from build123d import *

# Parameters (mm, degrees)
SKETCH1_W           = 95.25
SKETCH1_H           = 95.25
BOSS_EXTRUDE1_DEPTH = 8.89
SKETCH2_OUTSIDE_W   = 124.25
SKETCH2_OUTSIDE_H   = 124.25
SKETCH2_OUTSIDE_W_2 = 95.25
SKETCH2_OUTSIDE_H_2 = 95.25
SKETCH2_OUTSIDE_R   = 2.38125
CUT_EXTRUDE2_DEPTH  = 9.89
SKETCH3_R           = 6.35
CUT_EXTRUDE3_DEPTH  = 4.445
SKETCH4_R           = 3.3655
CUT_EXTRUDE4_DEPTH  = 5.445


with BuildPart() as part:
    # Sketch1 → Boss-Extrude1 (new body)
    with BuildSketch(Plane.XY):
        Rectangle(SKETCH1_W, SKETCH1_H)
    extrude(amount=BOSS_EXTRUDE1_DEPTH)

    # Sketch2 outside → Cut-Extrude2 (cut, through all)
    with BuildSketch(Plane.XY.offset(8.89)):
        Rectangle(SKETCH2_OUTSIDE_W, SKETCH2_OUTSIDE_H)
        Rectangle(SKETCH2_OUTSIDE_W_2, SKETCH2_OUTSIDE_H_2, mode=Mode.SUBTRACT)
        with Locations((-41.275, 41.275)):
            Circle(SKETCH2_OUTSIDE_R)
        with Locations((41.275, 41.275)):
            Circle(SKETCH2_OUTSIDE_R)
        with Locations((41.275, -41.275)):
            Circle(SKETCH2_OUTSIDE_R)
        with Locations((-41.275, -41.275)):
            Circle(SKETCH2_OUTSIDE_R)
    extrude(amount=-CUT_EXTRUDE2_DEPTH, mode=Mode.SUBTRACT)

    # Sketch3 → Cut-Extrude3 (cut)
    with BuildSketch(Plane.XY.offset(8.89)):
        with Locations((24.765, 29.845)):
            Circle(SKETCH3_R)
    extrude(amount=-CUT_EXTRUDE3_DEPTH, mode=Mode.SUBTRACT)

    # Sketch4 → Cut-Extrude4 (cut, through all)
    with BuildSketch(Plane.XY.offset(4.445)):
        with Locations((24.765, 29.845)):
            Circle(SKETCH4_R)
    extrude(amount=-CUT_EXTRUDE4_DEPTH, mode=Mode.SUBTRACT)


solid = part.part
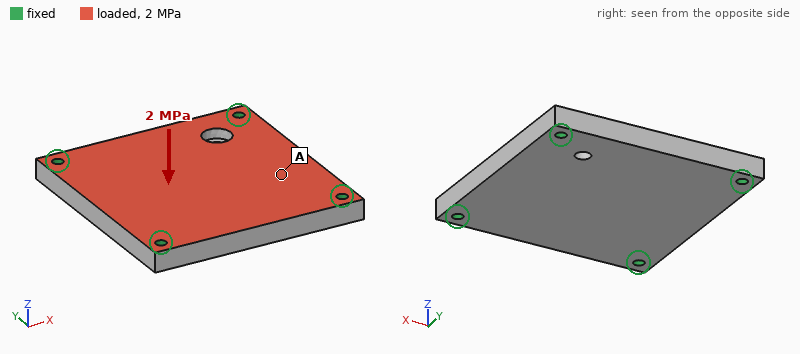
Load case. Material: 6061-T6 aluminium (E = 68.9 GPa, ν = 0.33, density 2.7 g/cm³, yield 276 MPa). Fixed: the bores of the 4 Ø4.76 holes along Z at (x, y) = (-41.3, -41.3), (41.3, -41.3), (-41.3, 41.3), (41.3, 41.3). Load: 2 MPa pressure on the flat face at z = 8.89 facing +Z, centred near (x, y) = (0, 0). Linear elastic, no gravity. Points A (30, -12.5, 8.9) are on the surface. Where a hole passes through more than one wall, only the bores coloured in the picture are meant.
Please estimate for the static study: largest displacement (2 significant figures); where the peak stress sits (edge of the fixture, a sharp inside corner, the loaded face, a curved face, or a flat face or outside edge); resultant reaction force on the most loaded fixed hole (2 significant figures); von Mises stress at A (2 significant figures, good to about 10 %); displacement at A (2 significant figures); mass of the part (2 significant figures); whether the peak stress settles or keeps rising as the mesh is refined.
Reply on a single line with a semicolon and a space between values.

0.19 mm; edge of the fixture; 4.5 kN; 45 MPa; 0.13 mm; 210 g; keeps rising
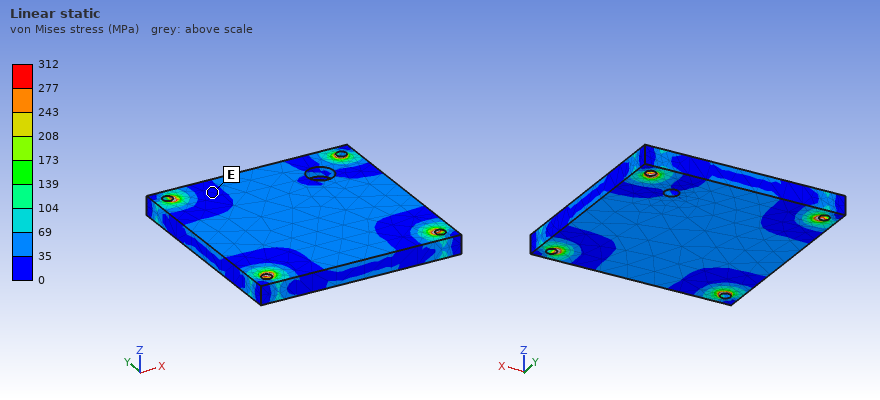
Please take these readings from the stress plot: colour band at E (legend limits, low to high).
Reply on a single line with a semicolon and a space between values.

0 to 35 MPa
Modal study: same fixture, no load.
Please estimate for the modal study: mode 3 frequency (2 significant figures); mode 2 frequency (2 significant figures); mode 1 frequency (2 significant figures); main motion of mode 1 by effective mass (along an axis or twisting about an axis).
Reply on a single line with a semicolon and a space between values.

6700 Hz; 6700 Hz; 3900 Hz; along Z
